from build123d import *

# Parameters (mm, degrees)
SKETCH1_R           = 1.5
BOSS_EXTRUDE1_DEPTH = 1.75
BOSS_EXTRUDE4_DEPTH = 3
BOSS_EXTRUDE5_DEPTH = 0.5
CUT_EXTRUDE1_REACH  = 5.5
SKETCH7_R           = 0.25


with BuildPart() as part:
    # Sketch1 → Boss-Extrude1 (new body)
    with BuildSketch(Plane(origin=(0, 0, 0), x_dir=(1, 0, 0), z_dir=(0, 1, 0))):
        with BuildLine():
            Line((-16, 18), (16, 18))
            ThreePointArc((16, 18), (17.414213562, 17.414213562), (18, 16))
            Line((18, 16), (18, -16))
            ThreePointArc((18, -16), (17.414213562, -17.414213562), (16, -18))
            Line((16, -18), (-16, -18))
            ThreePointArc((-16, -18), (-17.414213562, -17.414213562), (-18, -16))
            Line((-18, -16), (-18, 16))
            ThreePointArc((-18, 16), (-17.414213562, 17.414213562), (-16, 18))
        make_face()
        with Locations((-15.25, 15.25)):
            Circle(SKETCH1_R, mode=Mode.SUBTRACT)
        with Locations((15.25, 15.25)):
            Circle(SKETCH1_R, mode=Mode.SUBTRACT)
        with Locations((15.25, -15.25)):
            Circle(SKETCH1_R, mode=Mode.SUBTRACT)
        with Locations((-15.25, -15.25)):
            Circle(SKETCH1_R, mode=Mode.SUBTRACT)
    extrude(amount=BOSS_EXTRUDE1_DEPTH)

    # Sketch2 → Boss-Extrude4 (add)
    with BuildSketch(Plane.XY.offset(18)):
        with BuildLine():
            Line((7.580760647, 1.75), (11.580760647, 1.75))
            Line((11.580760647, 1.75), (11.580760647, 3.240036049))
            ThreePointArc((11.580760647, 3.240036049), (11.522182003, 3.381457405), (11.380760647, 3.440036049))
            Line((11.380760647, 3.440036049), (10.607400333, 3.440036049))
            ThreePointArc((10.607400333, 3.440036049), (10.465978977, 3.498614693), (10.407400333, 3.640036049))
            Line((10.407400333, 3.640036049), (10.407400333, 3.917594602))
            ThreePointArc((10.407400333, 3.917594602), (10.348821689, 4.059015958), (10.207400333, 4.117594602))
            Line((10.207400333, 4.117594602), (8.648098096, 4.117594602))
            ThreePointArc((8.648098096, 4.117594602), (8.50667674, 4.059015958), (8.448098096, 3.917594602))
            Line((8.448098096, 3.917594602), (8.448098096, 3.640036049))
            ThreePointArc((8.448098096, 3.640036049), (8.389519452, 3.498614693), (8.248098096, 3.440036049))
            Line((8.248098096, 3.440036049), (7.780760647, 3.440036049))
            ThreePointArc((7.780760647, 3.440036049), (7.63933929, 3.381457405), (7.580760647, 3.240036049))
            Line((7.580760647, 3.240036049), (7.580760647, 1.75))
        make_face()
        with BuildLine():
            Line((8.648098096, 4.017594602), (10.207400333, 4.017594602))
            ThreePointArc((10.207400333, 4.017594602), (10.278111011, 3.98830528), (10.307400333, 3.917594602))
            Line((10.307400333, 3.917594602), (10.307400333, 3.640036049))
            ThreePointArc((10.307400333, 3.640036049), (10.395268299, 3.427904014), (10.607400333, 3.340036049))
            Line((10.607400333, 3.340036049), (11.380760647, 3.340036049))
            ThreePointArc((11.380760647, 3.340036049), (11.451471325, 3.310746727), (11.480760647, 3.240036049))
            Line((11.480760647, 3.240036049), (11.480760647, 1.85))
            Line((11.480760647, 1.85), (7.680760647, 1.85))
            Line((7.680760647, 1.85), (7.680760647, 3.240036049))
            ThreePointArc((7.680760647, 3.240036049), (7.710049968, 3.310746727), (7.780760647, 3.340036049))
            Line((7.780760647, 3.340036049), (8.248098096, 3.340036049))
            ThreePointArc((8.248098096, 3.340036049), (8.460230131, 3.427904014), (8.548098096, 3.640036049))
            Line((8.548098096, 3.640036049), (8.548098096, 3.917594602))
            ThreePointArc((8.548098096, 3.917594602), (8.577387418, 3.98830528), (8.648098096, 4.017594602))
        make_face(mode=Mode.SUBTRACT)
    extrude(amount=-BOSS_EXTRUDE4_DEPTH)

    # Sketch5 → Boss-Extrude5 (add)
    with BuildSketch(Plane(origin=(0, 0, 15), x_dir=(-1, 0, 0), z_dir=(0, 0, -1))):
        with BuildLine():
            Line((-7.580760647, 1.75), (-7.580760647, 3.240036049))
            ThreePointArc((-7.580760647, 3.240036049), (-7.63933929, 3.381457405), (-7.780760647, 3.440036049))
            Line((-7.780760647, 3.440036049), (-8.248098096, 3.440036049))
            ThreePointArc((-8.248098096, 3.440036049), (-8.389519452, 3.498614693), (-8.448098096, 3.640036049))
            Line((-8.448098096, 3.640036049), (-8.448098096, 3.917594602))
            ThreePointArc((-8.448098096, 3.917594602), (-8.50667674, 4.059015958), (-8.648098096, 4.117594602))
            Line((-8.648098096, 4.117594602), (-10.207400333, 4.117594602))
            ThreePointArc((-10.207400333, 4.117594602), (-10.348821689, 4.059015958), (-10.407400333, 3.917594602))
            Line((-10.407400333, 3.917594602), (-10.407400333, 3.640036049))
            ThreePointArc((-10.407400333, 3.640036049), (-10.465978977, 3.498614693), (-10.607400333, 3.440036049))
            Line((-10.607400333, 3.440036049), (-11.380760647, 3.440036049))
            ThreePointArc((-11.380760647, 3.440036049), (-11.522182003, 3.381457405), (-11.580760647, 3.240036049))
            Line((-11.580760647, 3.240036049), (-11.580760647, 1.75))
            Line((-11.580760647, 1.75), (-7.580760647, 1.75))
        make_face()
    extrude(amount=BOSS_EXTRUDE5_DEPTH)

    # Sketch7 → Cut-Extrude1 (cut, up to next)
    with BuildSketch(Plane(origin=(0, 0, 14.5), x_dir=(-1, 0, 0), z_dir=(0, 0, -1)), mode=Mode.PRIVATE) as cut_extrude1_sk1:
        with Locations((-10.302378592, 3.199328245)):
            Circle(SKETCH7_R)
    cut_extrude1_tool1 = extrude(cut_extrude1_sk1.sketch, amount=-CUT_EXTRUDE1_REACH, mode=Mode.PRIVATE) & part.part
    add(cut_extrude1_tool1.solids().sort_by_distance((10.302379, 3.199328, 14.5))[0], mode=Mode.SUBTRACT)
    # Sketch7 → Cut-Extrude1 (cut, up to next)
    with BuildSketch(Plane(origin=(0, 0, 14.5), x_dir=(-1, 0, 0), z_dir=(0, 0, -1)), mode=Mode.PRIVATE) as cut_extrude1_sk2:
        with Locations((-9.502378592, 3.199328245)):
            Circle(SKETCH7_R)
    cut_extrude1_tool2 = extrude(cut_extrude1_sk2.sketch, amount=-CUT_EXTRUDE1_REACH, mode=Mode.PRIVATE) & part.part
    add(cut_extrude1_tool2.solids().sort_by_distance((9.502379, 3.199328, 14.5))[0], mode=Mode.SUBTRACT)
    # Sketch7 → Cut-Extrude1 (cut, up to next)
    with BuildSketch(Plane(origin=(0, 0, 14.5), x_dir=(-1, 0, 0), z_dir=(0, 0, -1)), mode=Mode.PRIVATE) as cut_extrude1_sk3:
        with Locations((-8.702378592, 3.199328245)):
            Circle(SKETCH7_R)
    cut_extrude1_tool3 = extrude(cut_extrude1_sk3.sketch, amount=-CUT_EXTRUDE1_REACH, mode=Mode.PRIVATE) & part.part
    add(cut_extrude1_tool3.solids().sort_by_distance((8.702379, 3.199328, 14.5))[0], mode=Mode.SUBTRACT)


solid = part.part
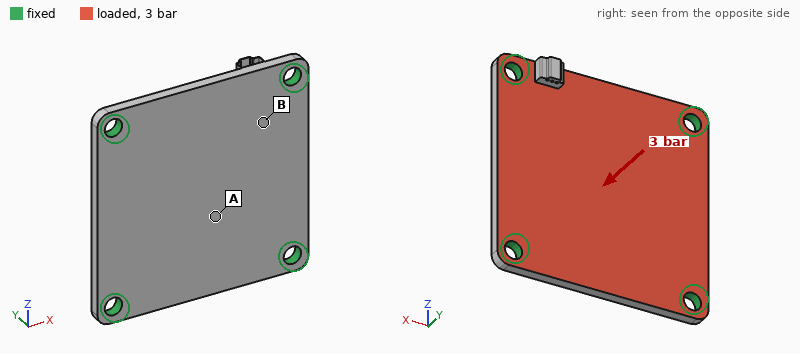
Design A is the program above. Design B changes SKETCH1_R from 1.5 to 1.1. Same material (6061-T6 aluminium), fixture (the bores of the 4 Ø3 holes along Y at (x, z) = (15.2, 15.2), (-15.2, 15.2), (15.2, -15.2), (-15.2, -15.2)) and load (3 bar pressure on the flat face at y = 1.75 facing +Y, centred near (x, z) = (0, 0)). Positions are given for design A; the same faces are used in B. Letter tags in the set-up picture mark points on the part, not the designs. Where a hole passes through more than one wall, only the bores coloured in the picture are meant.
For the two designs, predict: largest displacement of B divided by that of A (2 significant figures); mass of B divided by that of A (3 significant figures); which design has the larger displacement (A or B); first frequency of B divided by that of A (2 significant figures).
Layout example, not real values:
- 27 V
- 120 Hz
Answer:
- 1.1
- 1.01
- B
- 0.94
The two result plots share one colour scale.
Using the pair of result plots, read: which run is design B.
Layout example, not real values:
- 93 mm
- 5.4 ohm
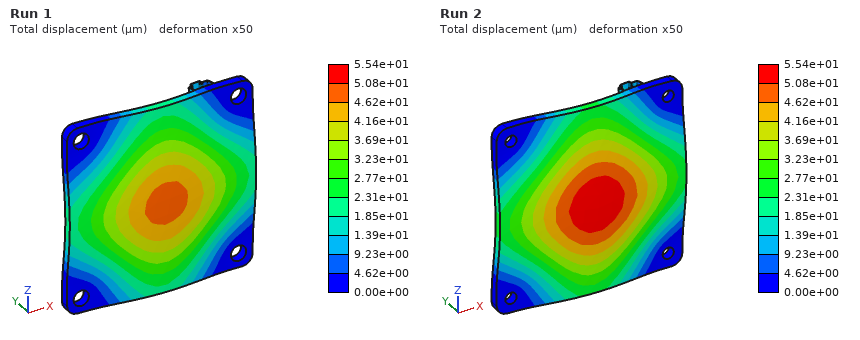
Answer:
- Run 2
